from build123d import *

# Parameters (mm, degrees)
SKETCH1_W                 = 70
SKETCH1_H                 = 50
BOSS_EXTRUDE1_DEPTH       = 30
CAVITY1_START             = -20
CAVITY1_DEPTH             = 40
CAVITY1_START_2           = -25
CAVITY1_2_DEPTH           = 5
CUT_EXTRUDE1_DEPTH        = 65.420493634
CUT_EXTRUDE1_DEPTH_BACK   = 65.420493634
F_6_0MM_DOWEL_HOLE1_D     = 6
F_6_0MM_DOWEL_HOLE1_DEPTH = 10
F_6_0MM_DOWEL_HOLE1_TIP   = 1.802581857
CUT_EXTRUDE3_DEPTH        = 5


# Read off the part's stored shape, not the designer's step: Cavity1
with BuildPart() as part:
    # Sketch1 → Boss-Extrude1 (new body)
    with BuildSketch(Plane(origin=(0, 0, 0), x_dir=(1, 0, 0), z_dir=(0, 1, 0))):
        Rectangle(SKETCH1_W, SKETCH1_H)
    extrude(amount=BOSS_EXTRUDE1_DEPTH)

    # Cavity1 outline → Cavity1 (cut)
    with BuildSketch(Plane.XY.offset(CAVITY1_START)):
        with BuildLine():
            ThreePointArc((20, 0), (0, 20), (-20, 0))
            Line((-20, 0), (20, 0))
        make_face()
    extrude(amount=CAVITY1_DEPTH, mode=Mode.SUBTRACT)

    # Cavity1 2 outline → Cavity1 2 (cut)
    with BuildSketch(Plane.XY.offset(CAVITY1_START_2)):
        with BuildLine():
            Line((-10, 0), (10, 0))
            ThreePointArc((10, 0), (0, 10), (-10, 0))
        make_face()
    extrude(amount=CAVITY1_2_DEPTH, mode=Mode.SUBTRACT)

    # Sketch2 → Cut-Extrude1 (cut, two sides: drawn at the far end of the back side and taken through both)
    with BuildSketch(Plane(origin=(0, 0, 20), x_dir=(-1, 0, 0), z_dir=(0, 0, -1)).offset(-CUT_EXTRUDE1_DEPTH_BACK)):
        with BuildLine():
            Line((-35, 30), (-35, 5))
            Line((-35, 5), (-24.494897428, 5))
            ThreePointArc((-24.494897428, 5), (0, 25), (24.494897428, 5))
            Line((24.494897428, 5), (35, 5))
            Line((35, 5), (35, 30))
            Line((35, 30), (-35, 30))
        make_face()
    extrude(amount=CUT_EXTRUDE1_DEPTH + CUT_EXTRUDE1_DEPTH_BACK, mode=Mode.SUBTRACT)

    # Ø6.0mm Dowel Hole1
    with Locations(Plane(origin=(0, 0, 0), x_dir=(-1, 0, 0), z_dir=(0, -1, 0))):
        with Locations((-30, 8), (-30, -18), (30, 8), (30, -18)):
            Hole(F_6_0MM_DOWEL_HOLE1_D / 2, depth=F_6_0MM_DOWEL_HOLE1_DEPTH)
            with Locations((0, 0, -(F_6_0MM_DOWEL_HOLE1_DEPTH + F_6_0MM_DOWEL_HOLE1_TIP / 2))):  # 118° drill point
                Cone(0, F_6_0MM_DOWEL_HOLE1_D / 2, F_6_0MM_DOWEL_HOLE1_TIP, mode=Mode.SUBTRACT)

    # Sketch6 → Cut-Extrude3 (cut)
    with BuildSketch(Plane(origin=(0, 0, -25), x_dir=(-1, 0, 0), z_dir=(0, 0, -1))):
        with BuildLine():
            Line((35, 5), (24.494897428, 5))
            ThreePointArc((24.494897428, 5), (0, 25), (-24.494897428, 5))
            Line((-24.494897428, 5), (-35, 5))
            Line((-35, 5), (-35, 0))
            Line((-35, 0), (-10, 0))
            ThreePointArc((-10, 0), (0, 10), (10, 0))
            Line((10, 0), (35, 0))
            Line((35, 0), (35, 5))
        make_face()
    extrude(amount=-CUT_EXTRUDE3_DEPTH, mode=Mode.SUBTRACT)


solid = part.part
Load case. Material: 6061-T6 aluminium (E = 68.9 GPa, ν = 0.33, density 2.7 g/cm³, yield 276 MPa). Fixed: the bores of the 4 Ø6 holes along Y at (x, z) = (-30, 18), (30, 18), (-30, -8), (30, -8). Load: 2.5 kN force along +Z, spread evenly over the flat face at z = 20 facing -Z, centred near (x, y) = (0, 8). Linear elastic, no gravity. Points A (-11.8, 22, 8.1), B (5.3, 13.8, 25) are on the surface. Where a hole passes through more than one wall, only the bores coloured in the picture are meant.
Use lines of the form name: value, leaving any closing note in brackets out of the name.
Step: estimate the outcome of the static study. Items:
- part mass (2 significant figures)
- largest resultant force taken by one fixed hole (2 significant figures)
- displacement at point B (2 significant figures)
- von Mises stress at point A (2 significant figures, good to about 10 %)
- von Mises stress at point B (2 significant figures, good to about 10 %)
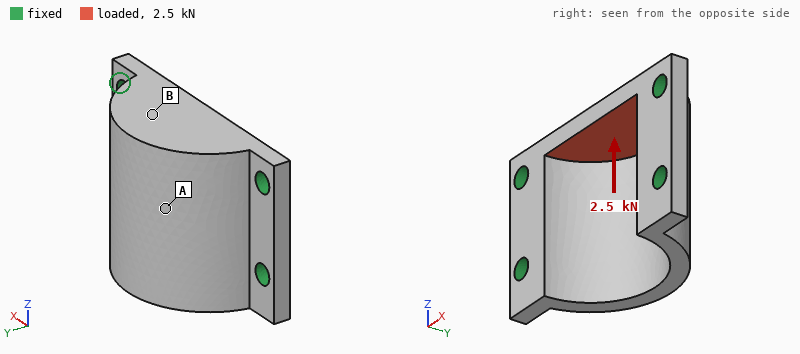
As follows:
part mass: 62 g
largest resultant force taken by one fixed hole: 750 N
displacement at point B: 21 µm
von Mises stress at point A: 6.1 MPa
von Mises stress at point B: 33 MPa
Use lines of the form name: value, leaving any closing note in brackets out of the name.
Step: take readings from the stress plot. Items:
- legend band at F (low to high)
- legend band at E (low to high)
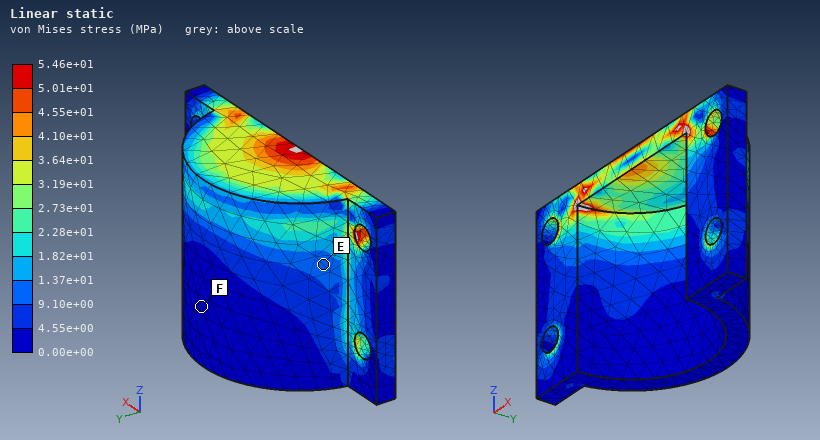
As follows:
legend band at F: 0.00e+00 to 4.55e+00 MPa
legend band at E: 9.10e+00 to 1.37e+01 MPa
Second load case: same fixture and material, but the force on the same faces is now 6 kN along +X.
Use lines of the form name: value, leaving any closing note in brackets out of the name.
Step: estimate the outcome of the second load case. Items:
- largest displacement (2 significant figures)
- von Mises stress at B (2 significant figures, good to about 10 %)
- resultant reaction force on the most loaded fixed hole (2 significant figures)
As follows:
largest displacement: 23 µm
von Mises stress at B: 18 MPa
resultant reaction force on the most loaded fixed hole: 2.8 kN
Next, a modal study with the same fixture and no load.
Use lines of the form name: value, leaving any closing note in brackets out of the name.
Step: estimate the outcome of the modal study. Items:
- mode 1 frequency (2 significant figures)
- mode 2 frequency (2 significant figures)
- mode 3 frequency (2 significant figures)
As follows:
mode 1 frequency: 10 kHz
mode 2 frequency: 10 kHz
mode 3 frequency: 15 kHz
